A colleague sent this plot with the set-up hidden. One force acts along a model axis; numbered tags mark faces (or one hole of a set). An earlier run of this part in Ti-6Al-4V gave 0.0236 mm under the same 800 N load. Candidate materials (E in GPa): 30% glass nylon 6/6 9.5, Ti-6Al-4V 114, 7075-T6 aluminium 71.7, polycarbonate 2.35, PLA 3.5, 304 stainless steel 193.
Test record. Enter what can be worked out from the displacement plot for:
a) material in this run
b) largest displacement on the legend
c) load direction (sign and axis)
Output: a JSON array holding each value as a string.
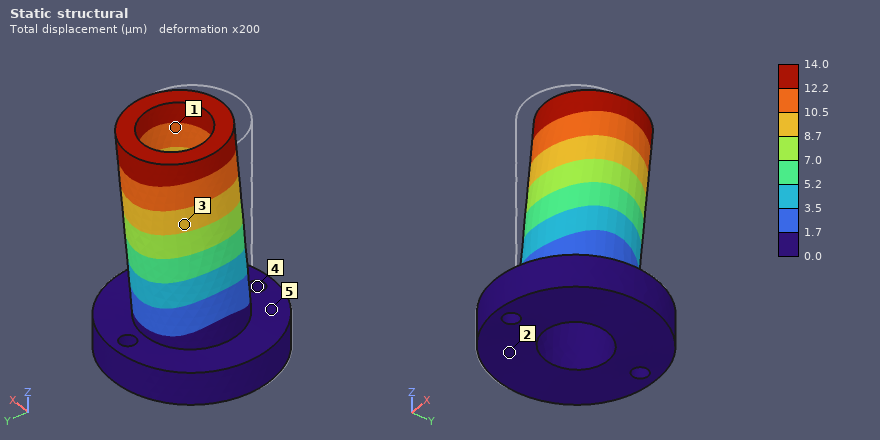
["304 stainless steel", "14.0 µm", "+Y"]
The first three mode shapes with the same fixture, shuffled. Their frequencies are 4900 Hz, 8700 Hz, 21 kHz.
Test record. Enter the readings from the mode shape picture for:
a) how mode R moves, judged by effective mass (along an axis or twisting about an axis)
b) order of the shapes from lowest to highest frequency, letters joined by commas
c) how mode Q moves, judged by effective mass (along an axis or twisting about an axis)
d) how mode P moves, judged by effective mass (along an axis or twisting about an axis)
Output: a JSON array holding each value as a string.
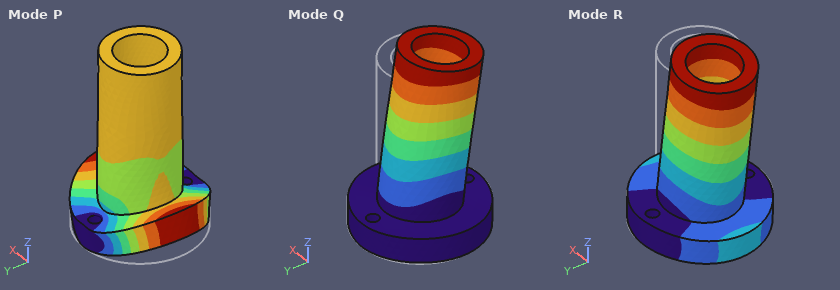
["along X", "R, Q, P", "along Y", "along Z"]
